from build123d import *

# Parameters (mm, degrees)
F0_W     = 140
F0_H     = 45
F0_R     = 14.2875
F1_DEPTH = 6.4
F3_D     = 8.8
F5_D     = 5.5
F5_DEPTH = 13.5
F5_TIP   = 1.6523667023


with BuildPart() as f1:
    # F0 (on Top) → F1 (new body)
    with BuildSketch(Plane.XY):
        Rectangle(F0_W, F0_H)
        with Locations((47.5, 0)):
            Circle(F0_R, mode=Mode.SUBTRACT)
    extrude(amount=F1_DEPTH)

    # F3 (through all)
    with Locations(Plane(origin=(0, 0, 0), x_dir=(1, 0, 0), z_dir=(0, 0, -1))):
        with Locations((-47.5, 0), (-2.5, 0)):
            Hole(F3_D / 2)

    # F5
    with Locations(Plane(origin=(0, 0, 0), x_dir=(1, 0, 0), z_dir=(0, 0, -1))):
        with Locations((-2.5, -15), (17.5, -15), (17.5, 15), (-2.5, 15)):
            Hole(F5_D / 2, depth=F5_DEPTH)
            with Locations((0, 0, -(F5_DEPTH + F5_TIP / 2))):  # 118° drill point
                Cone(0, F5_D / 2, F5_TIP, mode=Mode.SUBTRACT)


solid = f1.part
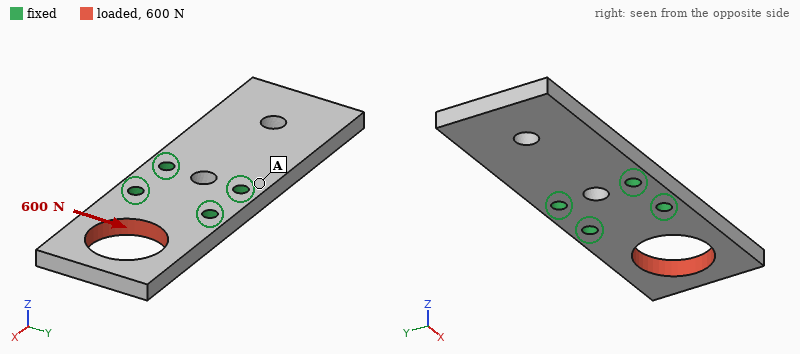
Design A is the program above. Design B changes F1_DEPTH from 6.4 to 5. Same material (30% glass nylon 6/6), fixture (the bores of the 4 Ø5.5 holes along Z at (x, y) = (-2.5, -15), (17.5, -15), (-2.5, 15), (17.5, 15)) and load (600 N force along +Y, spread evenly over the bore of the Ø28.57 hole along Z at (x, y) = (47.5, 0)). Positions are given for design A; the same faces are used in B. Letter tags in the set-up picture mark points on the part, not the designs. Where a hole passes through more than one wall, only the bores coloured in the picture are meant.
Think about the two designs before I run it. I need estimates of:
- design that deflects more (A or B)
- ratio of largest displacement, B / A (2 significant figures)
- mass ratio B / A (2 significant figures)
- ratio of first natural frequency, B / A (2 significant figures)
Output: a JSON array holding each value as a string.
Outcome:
["B", "1.3", "0.78", "0.79"]
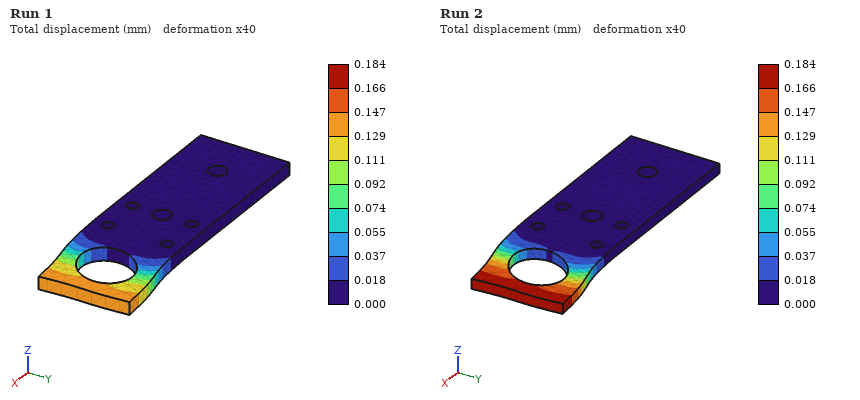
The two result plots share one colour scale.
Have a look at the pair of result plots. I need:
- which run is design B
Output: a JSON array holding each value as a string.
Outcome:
["Run 2"]
